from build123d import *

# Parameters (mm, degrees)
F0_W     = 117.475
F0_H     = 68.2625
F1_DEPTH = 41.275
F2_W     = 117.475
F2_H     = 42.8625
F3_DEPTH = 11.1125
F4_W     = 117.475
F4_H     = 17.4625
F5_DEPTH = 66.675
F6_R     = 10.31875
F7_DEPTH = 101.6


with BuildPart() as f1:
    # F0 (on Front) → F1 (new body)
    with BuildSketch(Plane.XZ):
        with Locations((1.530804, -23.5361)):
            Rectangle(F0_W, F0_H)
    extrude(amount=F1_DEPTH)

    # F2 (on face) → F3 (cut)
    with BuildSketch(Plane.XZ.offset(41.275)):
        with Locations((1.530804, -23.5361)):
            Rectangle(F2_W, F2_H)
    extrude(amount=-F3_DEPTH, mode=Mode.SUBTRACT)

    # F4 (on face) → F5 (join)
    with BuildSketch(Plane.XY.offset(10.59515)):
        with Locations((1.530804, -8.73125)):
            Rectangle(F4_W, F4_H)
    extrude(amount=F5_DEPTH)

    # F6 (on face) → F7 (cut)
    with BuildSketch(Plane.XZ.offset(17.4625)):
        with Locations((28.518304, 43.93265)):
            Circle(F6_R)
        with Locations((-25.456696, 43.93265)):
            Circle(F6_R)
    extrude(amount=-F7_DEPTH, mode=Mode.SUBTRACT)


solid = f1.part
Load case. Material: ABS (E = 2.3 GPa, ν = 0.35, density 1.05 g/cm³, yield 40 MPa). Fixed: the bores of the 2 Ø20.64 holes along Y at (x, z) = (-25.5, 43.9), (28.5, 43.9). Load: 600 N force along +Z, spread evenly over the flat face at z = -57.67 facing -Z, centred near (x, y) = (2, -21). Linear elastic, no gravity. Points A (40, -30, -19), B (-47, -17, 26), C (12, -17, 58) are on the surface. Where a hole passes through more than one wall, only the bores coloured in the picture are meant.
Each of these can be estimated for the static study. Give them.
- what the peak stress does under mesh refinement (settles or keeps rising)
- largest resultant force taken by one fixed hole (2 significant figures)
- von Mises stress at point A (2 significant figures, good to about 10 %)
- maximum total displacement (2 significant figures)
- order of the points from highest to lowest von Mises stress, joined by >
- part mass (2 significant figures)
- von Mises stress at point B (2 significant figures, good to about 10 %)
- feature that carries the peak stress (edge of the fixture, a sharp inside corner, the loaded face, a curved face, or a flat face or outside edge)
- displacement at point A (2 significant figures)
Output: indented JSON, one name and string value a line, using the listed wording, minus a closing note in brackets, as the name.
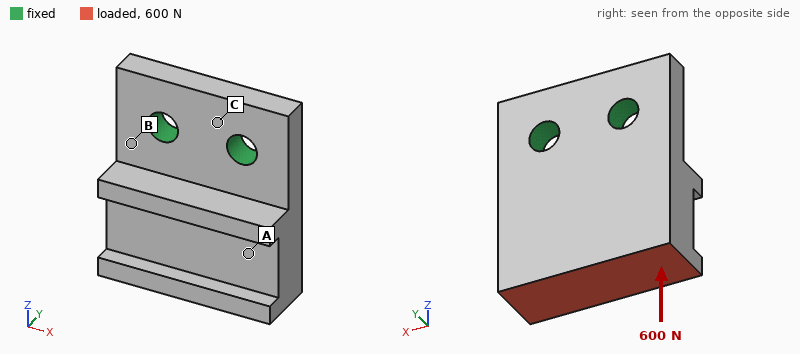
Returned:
{
  "what the peak stress does under mesh refinement": "keeps rising",
  "largest resultant force taken by one fixed hole": "300 N",
  "von Mises stress at point A": "0.34 MPa",
  "maximum total displacement": "0.19 mm",
  "order of the points from highest to lowest von Mises stress, joined by >": "B > A > C",
  "part mass": "420 g",
  "von Mises stress at point B": "1.1 MPa",
  "feature that carries the peak stress": "edge of the fixture",
  "displacement at point A": "0.097 mm"
}
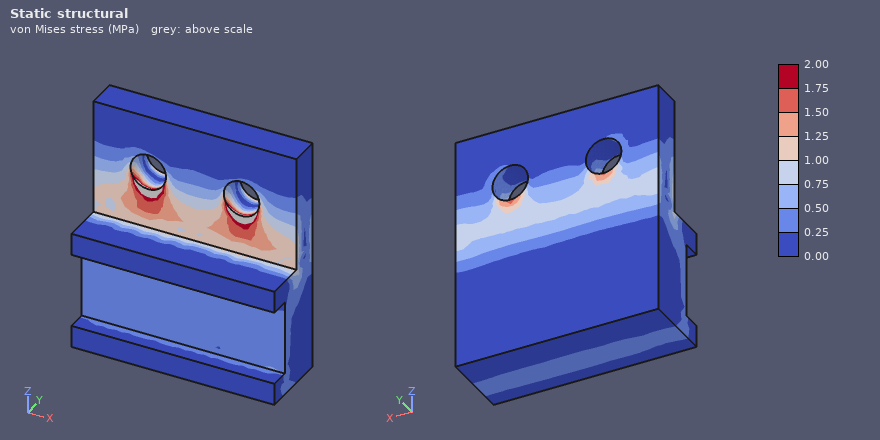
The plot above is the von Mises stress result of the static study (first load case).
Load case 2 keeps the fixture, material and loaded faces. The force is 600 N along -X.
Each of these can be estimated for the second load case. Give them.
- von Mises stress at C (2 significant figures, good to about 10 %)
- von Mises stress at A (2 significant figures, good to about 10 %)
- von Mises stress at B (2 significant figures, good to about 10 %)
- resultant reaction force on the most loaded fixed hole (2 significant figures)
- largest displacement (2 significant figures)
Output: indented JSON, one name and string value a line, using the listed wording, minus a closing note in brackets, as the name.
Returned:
{
  "von Mises stress at C": "0.28 MPa",
  "von Mises stress at A": "0.30 MPa",
  "von Mises stress at B": "0.83 MPa",
  "resultant reaction force on the most loaded fixed hole": "900 N",
  "largest displacement": "0.10 mm"
}
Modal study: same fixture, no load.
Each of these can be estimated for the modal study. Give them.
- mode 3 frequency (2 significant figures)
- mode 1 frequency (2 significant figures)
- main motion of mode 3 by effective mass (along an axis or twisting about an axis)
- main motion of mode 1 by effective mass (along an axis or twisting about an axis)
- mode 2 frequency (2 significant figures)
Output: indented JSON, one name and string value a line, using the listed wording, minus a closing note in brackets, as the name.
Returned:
{
  "mode 3 frequency": "1100 Hz",
  "mode 1 frequency": "330 Hz",
  "main motion of mode 3 by effective mass": "along X",
  "main motion of mode 1 by effective mass": "along Y",
  "mode 2 frequency": "840 Hz"
}
